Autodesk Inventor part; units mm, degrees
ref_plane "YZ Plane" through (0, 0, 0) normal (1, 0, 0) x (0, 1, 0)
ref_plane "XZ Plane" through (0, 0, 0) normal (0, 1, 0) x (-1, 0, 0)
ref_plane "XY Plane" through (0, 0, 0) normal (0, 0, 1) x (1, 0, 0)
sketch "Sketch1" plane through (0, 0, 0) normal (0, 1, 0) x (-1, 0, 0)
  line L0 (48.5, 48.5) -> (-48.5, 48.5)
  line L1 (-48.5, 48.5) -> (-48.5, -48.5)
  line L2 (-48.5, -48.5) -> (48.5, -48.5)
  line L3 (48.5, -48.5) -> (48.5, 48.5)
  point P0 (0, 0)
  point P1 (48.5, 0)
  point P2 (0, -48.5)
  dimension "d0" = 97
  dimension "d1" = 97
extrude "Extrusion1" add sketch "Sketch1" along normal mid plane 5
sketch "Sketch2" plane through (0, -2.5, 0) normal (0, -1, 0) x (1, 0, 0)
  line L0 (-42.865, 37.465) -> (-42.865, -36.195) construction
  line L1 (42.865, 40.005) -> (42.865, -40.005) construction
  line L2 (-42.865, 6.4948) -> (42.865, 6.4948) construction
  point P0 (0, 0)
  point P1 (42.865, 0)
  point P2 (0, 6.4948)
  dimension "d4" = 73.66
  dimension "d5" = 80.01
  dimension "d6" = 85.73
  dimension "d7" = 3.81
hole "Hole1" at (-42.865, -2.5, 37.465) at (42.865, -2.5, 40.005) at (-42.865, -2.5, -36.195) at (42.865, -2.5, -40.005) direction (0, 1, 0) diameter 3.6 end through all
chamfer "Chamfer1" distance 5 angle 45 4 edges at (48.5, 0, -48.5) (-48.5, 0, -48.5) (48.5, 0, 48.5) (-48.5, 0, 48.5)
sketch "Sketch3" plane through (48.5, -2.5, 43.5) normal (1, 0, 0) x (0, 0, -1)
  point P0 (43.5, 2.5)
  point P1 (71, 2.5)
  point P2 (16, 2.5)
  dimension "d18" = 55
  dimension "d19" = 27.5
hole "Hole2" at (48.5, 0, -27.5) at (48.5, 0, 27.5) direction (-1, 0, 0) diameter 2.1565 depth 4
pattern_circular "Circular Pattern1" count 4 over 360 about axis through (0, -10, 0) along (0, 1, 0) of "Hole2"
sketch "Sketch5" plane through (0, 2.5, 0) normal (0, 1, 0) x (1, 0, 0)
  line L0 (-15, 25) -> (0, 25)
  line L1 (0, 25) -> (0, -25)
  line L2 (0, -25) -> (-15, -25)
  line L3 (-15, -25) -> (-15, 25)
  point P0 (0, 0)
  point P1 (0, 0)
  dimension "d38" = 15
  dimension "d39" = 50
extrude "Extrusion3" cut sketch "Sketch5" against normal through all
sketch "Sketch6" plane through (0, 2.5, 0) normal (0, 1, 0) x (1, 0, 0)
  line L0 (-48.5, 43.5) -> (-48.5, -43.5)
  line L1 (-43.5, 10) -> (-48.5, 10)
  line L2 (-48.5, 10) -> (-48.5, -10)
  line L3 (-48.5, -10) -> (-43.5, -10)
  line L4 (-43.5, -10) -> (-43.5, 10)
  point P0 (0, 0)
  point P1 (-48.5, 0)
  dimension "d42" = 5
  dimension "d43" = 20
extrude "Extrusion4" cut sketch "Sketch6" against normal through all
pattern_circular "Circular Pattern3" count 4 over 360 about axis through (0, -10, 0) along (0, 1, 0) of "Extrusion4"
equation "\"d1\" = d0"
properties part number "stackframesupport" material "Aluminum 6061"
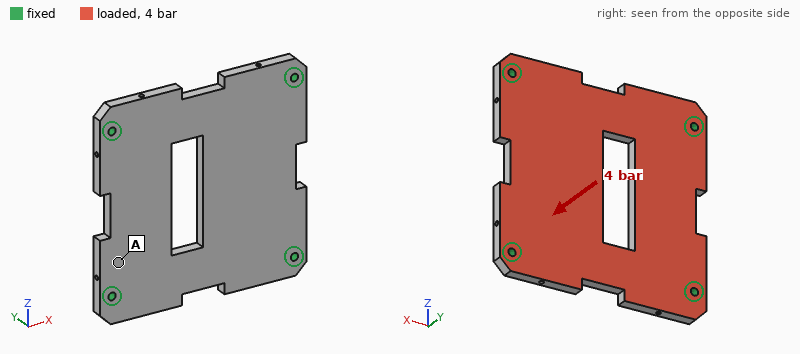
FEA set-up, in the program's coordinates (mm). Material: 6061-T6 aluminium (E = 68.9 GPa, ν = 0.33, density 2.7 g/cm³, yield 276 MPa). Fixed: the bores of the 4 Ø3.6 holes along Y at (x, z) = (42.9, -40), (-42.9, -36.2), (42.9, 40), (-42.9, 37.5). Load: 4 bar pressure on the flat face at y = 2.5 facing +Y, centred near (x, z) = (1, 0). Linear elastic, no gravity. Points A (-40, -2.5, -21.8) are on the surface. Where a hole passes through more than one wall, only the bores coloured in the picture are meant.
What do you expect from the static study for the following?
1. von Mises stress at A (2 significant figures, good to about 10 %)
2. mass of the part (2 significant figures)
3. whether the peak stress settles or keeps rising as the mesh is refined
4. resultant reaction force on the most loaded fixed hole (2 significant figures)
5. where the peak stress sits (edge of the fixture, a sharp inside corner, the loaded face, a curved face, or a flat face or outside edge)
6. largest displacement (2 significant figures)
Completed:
23 MPa
110 g
keeps rising
830 N
edge of the fixture
0.27 mm
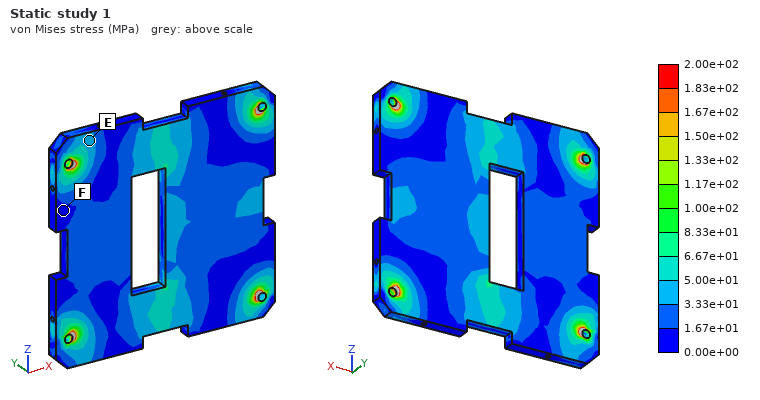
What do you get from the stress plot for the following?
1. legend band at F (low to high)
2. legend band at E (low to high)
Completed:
0.00e+00 to 1.67e+01 MPa
3.33e+01 to 5.00e+01 MPa
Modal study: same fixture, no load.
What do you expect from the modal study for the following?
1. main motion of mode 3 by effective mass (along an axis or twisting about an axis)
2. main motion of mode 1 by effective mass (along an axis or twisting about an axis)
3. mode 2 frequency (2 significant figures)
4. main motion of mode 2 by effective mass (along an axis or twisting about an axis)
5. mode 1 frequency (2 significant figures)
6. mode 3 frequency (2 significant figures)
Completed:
twisting about Z
along Y
3800 Hz
twisting about X
2300 Hz
4000 Hz
